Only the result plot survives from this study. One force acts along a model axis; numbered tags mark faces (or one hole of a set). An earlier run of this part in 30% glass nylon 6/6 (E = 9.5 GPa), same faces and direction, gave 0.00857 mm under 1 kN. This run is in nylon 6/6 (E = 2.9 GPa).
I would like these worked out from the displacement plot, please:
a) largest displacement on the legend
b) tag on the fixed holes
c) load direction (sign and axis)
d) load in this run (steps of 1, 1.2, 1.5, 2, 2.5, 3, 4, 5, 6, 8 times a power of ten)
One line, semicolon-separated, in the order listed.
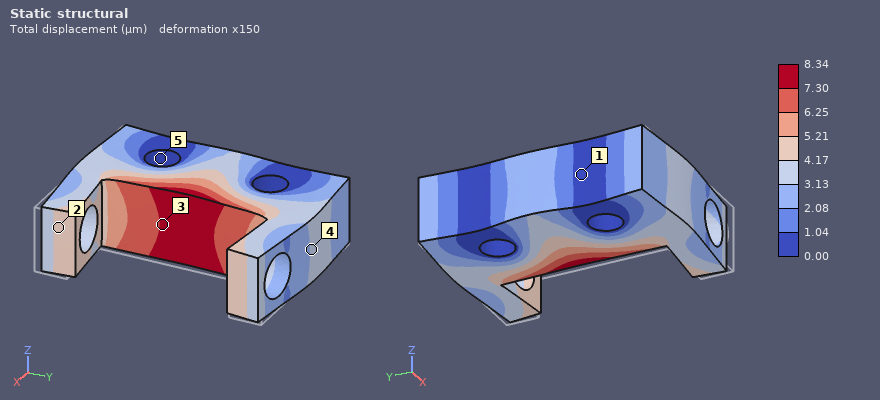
8.34 µm; 5; -X; 300 N
